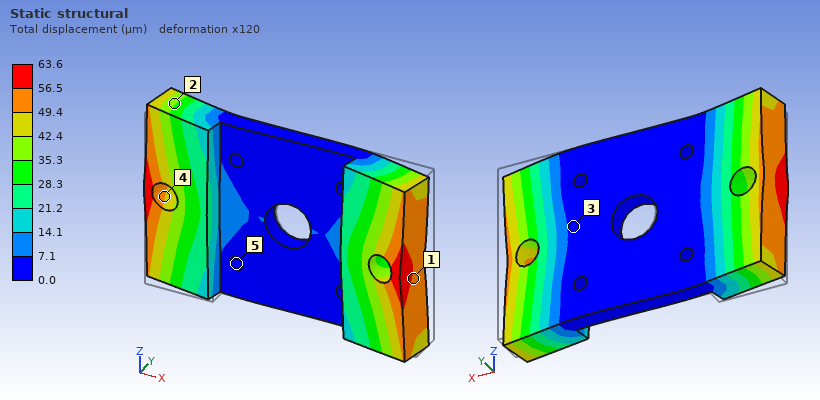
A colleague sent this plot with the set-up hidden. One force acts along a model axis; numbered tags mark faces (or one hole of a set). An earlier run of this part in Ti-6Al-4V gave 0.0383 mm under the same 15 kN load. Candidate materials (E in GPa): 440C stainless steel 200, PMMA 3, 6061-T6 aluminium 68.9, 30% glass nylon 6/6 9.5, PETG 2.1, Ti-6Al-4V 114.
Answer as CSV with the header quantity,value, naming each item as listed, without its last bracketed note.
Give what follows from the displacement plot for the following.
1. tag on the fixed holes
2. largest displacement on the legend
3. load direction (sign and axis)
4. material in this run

quantity,value
tag on the fixed holes,5
largest displacement on the legend,63.6 µm
load direction,-X
material in this run,6061-T6 aluminium
